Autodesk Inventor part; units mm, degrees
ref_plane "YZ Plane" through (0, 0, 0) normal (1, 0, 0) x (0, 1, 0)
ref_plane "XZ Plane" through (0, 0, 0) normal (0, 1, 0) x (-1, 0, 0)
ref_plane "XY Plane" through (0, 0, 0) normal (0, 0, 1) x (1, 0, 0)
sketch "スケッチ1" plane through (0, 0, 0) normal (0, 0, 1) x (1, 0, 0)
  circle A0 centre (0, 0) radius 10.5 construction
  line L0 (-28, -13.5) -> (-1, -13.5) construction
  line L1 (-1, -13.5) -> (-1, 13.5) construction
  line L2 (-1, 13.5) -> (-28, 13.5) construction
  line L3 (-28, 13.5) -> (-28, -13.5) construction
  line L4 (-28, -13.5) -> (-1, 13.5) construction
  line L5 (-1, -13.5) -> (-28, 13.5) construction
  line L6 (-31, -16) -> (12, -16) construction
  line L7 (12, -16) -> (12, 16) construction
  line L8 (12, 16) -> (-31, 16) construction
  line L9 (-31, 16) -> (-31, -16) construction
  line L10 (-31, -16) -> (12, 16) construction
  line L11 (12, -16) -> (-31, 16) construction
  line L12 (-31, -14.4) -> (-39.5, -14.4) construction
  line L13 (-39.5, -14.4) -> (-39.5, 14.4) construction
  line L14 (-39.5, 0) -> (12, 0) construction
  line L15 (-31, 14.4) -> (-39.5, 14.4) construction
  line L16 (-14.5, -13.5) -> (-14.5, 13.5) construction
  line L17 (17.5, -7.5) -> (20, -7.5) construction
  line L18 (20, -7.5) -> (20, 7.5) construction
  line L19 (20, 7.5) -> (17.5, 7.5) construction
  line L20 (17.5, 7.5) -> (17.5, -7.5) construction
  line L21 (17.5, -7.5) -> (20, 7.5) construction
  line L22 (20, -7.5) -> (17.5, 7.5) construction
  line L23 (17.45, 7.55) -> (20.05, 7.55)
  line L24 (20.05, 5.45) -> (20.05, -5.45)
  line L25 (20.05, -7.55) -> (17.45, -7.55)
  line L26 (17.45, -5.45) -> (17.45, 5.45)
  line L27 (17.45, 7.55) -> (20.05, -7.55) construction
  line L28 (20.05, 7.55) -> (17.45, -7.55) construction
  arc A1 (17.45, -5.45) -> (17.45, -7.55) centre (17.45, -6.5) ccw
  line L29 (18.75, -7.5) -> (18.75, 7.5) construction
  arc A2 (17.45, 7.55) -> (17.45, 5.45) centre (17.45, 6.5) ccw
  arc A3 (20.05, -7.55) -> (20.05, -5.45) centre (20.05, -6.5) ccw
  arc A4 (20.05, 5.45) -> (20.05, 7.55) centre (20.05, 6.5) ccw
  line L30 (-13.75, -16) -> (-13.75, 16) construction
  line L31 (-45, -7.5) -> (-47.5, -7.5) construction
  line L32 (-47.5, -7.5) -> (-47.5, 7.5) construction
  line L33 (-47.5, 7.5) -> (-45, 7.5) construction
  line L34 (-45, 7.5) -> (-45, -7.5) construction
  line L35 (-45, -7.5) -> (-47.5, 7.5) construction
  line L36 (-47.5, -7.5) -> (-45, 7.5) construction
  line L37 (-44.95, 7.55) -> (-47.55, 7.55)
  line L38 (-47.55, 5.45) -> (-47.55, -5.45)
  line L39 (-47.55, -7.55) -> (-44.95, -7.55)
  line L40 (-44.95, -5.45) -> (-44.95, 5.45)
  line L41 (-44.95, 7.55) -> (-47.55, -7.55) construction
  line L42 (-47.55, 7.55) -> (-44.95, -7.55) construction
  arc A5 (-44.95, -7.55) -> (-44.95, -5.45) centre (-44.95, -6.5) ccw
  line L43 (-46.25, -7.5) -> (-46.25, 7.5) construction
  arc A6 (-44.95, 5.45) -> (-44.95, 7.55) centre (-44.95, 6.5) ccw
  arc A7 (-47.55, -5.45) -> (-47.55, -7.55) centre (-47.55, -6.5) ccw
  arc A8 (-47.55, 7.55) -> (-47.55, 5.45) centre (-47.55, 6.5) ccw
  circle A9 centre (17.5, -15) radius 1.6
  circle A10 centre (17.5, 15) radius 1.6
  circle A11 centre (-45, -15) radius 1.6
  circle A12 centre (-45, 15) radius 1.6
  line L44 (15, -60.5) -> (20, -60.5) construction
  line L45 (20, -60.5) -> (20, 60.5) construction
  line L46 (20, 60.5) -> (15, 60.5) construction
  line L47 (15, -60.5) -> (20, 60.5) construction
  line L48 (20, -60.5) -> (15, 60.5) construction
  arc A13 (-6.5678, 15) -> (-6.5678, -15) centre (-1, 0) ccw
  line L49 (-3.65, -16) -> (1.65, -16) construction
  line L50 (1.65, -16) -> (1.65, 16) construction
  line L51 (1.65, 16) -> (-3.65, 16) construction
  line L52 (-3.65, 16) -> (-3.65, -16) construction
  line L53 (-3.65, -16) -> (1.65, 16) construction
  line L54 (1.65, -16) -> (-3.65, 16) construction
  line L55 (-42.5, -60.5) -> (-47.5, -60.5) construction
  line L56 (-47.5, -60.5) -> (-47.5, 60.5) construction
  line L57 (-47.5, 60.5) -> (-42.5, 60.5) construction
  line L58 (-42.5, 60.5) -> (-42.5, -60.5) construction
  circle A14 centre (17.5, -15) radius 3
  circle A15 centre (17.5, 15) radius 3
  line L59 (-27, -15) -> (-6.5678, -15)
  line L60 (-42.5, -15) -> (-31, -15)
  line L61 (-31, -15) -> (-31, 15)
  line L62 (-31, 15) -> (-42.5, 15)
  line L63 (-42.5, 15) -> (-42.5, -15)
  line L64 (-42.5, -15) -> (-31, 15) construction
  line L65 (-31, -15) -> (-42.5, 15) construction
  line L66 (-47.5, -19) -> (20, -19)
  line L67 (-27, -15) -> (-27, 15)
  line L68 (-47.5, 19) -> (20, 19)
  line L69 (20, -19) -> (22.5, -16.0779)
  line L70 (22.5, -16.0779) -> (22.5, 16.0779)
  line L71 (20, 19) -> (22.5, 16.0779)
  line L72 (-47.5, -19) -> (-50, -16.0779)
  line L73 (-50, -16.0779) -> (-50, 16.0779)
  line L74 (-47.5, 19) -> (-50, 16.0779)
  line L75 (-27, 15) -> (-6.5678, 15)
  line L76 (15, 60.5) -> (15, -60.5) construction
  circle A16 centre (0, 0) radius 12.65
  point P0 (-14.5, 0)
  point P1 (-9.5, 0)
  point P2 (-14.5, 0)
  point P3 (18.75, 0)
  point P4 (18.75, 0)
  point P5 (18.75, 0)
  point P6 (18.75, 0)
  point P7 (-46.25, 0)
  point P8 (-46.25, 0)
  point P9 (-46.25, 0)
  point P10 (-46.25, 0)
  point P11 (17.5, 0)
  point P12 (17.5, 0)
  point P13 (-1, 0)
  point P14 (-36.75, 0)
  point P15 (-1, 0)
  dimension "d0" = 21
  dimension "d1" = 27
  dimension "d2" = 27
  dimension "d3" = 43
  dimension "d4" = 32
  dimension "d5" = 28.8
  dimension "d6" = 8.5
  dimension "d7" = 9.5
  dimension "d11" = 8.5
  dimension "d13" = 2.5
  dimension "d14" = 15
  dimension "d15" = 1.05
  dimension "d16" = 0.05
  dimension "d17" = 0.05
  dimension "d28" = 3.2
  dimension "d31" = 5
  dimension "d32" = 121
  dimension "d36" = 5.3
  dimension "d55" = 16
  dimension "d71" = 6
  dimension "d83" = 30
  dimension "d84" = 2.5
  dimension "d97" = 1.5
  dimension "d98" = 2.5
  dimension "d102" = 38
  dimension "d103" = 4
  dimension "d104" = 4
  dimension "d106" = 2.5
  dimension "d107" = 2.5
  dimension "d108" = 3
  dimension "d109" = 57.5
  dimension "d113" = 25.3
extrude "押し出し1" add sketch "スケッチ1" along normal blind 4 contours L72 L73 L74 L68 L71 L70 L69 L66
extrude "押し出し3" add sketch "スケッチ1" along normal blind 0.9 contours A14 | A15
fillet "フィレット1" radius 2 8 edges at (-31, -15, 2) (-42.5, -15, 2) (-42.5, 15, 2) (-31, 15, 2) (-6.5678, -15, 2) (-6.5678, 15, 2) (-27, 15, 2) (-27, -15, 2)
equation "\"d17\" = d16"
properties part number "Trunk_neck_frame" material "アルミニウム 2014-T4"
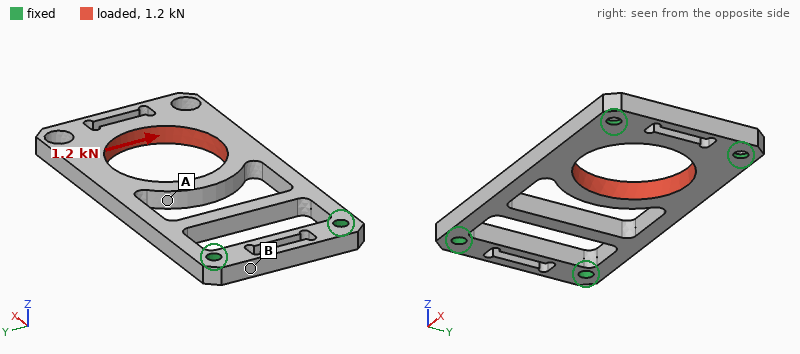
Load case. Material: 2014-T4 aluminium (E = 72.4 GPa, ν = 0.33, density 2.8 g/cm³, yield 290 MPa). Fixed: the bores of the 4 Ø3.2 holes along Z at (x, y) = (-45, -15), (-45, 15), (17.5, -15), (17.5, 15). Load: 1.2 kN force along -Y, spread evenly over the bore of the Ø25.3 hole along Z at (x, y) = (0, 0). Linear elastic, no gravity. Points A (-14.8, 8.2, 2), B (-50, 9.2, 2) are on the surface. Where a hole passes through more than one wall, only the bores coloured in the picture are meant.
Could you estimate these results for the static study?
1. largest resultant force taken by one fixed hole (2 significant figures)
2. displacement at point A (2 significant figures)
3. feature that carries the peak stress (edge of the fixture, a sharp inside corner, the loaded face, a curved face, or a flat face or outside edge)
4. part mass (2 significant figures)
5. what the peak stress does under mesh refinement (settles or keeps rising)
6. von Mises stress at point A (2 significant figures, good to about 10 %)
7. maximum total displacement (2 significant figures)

560 N
65 µm
edge of the fixture
15 g
keeps rising
28 MPa
67 µm
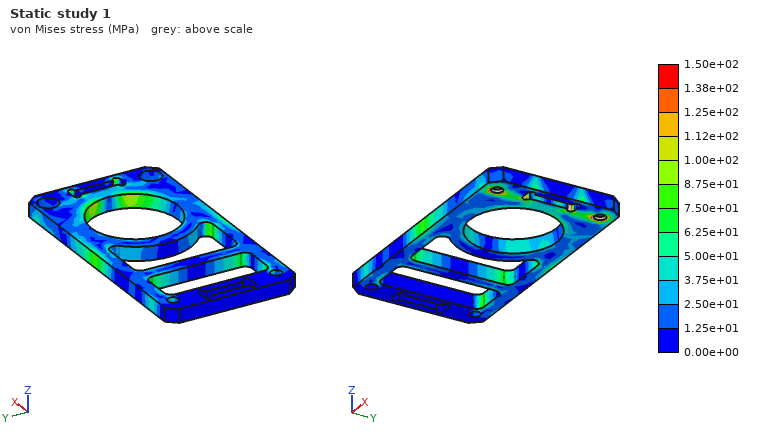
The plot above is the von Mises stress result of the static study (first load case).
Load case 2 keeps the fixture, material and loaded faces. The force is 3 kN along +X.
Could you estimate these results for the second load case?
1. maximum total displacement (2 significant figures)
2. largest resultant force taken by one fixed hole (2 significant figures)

68 µm
1.0 kN
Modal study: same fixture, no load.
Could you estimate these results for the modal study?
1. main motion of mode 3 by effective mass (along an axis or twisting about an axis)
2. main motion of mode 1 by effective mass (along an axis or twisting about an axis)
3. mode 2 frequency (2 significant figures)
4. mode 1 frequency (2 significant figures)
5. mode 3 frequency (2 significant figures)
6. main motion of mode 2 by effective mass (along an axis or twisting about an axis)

along Y
along Z
5400 Hz
3500 Hz
7400 Hz
twisting about X
